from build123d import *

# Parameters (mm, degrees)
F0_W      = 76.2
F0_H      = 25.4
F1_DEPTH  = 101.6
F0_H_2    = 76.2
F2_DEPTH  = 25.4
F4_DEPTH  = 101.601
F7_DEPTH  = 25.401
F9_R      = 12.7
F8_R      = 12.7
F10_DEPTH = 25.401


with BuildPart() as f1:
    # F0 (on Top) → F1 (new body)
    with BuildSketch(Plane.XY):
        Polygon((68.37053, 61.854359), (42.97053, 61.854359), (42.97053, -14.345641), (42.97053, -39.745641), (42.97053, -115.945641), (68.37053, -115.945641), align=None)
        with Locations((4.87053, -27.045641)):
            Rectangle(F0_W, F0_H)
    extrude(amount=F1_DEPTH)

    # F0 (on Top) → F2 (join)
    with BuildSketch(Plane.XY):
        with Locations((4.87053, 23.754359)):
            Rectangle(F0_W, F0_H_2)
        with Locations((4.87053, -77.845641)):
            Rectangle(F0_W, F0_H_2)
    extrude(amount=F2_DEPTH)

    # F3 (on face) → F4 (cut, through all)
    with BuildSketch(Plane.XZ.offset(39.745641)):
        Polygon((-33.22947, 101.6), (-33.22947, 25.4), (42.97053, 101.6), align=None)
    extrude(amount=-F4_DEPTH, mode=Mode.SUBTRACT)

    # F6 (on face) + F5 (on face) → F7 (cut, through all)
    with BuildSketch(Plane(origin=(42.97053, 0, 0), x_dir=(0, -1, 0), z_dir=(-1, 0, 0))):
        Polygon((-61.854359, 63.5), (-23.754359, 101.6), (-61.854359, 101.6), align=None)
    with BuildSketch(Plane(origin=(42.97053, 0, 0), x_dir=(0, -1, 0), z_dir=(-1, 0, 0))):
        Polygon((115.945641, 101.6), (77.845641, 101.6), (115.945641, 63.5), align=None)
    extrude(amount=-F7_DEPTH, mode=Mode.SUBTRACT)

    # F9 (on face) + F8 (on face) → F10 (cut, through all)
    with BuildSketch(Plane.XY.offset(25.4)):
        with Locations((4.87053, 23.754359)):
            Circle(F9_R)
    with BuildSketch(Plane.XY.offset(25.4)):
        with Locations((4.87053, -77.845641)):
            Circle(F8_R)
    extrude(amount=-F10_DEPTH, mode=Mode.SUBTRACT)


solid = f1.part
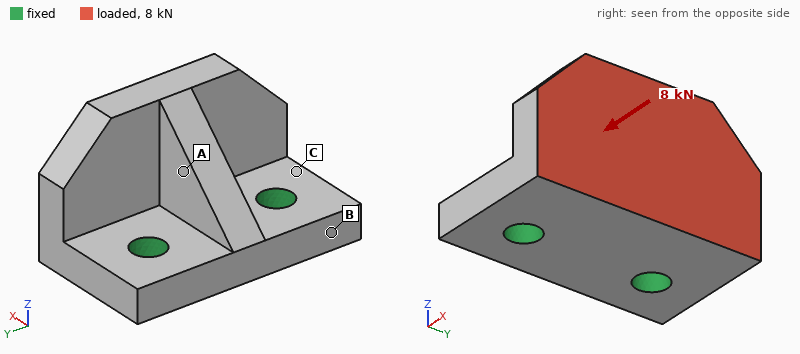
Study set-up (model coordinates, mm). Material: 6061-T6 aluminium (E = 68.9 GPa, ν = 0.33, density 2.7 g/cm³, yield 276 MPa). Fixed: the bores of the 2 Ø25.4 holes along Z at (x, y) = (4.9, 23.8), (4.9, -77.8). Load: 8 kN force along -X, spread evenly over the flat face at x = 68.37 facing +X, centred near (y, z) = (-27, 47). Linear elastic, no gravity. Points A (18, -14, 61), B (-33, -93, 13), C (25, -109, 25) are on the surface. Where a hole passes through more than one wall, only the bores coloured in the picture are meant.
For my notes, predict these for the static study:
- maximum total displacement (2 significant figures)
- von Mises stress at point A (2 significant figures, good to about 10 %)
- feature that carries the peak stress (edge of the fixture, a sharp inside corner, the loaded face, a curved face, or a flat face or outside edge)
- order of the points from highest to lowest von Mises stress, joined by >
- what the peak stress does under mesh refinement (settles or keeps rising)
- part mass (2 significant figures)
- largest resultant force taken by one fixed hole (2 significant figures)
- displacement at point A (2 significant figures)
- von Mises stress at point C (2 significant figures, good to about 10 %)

42 µm
4.1 MPa
edge of the fixture
C > A > B
keeps rising
2.2 kg
4.0 kN
18 µm
7.4 MPa
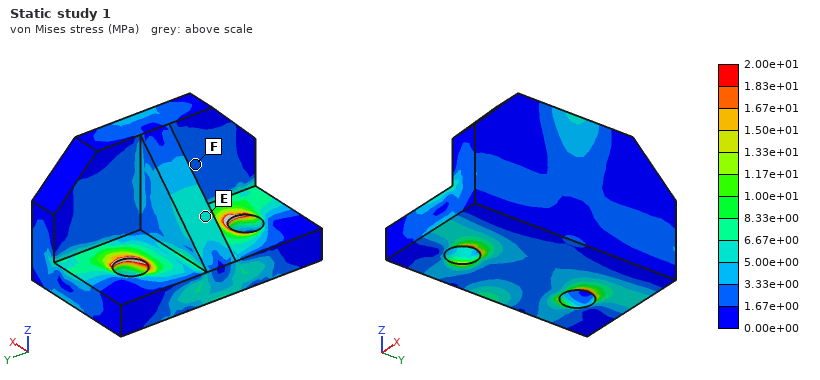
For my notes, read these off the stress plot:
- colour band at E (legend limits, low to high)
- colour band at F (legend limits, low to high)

5.00e+00 to 6.67e+00 MPa
1.67e+00 to 3.33e+00 MPa
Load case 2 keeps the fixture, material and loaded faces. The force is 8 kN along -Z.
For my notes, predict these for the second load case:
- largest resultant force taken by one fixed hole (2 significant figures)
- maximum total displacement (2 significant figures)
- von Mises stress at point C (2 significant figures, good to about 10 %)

4.0 kN
55 µm
9.8 MPa
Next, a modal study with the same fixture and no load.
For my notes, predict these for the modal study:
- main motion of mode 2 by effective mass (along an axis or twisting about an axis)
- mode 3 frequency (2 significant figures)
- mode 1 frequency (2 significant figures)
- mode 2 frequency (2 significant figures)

along Y
4600 Hz
2100 Hz
3100 Hz
